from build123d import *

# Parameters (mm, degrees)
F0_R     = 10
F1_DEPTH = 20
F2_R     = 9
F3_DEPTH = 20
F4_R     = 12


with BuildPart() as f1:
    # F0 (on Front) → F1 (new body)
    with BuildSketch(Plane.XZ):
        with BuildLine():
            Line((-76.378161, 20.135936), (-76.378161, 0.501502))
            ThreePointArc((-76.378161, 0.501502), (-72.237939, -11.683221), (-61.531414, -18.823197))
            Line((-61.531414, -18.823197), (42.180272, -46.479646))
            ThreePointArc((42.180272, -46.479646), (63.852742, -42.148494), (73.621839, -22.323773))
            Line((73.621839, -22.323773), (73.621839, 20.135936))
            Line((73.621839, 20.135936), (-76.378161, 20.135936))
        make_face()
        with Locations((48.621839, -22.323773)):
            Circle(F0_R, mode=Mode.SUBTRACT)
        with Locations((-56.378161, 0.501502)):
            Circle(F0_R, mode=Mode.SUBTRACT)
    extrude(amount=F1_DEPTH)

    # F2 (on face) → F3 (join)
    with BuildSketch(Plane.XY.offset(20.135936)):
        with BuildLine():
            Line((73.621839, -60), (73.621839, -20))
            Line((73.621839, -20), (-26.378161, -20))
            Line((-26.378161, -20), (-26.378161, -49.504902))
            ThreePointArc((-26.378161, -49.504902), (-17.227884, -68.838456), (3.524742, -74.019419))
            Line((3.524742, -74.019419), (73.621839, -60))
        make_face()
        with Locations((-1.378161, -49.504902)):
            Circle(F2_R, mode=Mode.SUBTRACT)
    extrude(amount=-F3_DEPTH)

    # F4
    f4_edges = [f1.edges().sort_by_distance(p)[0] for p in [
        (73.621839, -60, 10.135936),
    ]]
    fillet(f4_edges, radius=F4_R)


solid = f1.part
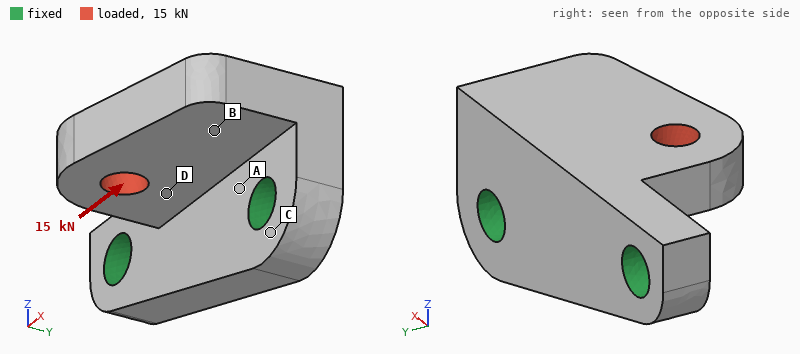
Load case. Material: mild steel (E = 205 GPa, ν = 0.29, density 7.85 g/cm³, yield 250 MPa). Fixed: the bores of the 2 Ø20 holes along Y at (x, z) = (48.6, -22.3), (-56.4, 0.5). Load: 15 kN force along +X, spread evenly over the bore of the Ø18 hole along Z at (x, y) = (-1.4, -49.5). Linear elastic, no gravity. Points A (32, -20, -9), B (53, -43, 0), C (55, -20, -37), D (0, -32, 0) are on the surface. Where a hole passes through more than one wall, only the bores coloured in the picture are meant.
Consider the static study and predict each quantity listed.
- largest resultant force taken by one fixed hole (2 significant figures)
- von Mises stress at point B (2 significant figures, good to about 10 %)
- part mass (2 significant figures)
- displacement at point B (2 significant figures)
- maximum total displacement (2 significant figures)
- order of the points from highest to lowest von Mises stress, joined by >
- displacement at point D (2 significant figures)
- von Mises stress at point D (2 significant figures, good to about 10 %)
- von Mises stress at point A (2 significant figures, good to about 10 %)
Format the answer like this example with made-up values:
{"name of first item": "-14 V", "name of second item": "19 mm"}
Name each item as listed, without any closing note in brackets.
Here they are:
{"largest resultant force taken by one fixed hole": "10.0 kN", "von Mises stress at point B": "13 MPa", "part mass": "1.9 kg", "displacement at point B": "13 µm", "maximum total displacement": "20 µm", "order of the points from highest to lowest von Mises stress, joined by >": "D > A > B > C", "displacement at point D": "8.4 µm", "von Mises stress at point D": "35 MPa", "von Mises stress at point A": "24 MPa"}
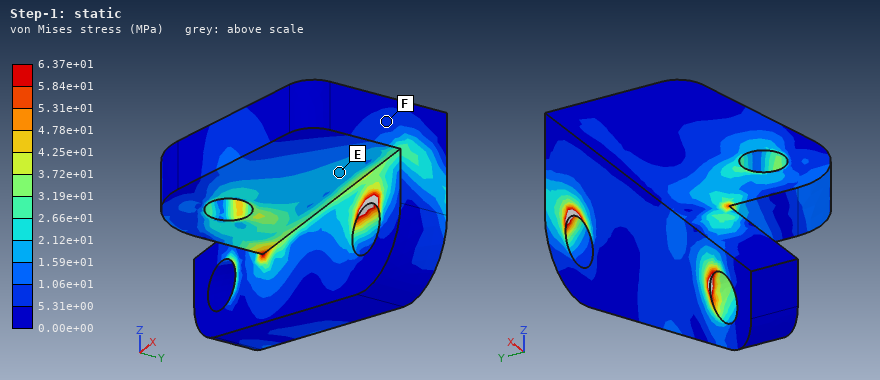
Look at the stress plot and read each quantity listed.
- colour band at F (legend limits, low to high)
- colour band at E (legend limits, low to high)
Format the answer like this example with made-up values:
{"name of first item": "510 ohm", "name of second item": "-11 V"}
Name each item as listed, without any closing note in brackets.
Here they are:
{"colour band at F": "5.31e+00 to 1.06e+01 MPa", "colour band at E": "1.59e+01 to 2.12e+01 MPa"}
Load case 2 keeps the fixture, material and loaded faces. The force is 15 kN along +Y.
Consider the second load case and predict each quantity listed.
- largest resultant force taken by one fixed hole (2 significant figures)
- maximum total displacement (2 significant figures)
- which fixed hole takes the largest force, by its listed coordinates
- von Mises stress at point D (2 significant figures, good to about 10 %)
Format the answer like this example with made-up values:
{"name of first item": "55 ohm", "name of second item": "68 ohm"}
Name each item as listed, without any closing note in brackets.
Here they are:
{"largest resultant force taken by one fixed hole": "8.5 kN", "maximum total displacement": "32 µm", "which fixed hole takes the largest force, by its listed coordinates": "(-56.4, 0.5)", "von Mises stress at point D": "14 MPa"}
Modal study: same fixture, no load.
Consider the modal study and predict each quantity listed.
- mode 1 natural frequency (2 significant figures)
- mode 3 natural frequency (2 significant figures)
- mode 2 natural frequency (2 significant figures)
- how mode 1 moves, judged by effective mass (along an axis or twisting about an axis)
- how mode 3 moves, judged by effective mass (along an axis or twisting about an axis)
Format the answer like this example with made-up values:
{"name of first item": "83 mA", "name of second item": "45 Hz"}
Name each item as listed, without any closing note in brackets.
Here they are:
{"mode 1 natural frequency": "2900 Hz", "mode 3 natural frequency": "6500 Hz", "mode 2 natural frequency": "5700 Hz", "how mode 1 moves, judged by effective mass": "along Z", "how mode 3 moves, judged by effective mass": "along Y"}
